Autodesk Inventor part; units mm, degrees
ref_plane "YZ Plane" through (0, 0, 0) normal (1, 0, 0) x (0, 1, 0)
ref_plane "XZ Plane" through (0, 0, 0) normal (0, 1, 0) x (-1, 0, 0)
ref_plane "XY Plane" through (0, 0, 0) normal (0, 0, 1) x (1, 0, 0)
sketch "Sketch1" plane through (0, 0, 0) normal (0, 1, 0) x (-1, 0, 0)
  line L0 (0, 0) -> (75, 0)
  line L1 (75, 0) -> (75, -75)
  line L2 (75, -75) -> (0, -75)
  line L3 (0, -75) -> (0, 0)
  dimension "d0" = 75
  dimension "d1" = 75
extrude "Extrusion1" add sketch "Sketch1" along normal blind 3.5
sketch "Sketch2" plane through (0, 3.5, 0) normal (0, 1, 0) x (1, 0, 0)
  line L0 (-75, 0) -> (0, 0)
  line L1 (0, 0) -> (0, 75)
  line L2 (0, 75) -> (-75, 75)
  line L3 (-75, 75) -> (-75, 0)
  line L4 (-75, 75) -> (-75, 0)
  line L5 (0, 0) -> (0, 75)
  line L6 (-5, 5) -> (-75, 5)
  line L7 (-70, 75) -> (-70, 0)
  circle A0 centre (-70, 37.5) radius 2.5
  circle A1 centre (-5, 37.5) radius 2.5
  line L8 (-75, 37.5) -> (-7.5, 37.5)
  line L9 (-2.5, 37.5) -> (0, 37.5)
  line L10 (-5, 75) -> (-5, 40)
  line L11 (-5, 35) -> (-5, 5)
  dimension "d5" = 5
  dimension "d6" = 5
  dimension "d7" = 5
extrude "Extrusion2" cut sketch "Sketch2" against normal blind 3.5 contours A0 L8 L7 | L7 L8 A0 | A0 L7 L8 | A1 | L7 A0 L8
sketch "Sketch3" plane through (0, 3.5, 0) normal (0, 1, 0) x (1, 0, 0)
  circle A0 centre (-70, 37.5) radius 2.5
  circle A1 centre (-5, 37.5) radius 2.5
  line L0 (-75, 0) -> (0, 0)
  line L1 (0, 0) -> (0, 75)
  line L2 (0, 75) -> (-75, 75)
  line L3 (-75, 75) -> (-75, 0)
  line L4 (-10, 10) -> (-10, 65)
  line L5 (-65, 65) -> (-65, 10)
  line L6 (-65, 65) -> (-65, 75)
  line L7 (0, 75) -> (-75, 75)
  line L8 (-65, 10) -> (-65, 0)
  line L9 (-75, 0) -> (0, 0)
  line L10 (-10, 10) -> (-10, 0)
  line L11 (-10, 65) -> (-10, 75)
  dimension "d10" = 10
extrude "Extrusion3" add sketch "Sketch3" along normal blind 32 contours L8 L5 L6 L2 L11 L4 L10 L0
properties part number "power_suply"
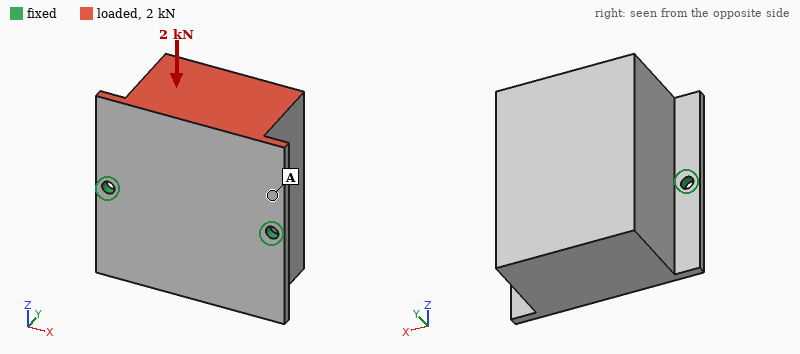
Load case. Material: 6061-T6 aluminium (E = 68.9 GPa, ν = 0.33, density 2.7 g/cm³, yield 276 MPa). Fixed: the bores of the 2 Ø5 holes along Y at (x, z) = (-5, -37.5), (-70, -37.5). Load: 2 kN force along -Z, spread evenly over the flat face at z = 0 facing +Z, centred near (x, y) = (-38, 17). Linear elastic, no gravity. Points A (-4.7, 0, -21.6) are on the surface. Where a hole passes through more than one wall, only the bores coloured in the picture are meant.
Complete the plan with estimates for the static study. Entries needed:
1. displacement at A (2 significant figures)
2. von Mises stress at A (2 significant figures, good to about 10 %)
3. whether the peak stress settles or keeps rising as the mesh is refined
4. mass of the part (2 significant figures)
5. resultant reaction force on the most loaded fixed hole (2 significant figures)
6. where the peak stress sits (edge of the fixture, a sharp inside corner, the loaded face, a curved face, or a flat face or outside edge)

0.098 mm
31 MPa
keeps rising
410 g
1.0 kN
edge of the fixture
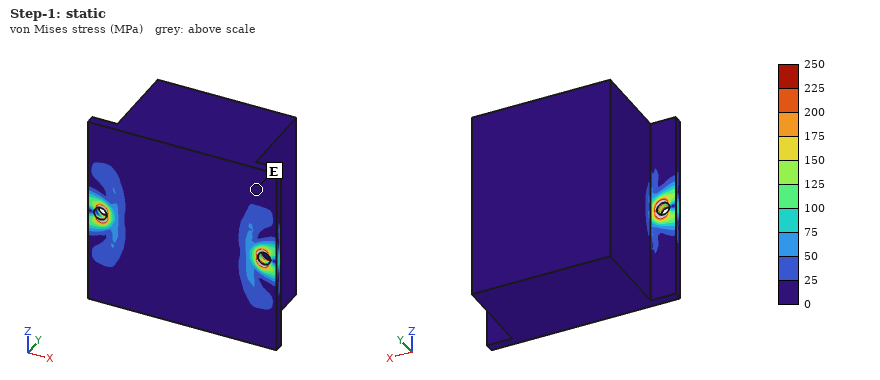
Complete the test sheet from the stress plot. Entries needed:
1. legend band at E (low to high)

0 to 25 MPa
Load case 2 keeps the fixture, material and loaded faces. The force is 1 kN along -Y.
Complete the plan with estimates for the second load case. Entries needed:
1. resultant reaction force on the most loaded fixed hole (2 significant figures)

570 N
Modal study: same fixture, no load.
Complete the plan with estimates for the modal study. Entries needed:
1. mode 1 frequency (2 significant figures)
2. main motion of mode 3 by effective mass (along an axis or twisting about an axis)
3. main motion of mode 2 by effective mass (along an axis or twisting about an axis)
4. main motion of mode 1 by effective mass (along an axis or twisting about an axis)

580 Hz
along X
along Y
along Z
